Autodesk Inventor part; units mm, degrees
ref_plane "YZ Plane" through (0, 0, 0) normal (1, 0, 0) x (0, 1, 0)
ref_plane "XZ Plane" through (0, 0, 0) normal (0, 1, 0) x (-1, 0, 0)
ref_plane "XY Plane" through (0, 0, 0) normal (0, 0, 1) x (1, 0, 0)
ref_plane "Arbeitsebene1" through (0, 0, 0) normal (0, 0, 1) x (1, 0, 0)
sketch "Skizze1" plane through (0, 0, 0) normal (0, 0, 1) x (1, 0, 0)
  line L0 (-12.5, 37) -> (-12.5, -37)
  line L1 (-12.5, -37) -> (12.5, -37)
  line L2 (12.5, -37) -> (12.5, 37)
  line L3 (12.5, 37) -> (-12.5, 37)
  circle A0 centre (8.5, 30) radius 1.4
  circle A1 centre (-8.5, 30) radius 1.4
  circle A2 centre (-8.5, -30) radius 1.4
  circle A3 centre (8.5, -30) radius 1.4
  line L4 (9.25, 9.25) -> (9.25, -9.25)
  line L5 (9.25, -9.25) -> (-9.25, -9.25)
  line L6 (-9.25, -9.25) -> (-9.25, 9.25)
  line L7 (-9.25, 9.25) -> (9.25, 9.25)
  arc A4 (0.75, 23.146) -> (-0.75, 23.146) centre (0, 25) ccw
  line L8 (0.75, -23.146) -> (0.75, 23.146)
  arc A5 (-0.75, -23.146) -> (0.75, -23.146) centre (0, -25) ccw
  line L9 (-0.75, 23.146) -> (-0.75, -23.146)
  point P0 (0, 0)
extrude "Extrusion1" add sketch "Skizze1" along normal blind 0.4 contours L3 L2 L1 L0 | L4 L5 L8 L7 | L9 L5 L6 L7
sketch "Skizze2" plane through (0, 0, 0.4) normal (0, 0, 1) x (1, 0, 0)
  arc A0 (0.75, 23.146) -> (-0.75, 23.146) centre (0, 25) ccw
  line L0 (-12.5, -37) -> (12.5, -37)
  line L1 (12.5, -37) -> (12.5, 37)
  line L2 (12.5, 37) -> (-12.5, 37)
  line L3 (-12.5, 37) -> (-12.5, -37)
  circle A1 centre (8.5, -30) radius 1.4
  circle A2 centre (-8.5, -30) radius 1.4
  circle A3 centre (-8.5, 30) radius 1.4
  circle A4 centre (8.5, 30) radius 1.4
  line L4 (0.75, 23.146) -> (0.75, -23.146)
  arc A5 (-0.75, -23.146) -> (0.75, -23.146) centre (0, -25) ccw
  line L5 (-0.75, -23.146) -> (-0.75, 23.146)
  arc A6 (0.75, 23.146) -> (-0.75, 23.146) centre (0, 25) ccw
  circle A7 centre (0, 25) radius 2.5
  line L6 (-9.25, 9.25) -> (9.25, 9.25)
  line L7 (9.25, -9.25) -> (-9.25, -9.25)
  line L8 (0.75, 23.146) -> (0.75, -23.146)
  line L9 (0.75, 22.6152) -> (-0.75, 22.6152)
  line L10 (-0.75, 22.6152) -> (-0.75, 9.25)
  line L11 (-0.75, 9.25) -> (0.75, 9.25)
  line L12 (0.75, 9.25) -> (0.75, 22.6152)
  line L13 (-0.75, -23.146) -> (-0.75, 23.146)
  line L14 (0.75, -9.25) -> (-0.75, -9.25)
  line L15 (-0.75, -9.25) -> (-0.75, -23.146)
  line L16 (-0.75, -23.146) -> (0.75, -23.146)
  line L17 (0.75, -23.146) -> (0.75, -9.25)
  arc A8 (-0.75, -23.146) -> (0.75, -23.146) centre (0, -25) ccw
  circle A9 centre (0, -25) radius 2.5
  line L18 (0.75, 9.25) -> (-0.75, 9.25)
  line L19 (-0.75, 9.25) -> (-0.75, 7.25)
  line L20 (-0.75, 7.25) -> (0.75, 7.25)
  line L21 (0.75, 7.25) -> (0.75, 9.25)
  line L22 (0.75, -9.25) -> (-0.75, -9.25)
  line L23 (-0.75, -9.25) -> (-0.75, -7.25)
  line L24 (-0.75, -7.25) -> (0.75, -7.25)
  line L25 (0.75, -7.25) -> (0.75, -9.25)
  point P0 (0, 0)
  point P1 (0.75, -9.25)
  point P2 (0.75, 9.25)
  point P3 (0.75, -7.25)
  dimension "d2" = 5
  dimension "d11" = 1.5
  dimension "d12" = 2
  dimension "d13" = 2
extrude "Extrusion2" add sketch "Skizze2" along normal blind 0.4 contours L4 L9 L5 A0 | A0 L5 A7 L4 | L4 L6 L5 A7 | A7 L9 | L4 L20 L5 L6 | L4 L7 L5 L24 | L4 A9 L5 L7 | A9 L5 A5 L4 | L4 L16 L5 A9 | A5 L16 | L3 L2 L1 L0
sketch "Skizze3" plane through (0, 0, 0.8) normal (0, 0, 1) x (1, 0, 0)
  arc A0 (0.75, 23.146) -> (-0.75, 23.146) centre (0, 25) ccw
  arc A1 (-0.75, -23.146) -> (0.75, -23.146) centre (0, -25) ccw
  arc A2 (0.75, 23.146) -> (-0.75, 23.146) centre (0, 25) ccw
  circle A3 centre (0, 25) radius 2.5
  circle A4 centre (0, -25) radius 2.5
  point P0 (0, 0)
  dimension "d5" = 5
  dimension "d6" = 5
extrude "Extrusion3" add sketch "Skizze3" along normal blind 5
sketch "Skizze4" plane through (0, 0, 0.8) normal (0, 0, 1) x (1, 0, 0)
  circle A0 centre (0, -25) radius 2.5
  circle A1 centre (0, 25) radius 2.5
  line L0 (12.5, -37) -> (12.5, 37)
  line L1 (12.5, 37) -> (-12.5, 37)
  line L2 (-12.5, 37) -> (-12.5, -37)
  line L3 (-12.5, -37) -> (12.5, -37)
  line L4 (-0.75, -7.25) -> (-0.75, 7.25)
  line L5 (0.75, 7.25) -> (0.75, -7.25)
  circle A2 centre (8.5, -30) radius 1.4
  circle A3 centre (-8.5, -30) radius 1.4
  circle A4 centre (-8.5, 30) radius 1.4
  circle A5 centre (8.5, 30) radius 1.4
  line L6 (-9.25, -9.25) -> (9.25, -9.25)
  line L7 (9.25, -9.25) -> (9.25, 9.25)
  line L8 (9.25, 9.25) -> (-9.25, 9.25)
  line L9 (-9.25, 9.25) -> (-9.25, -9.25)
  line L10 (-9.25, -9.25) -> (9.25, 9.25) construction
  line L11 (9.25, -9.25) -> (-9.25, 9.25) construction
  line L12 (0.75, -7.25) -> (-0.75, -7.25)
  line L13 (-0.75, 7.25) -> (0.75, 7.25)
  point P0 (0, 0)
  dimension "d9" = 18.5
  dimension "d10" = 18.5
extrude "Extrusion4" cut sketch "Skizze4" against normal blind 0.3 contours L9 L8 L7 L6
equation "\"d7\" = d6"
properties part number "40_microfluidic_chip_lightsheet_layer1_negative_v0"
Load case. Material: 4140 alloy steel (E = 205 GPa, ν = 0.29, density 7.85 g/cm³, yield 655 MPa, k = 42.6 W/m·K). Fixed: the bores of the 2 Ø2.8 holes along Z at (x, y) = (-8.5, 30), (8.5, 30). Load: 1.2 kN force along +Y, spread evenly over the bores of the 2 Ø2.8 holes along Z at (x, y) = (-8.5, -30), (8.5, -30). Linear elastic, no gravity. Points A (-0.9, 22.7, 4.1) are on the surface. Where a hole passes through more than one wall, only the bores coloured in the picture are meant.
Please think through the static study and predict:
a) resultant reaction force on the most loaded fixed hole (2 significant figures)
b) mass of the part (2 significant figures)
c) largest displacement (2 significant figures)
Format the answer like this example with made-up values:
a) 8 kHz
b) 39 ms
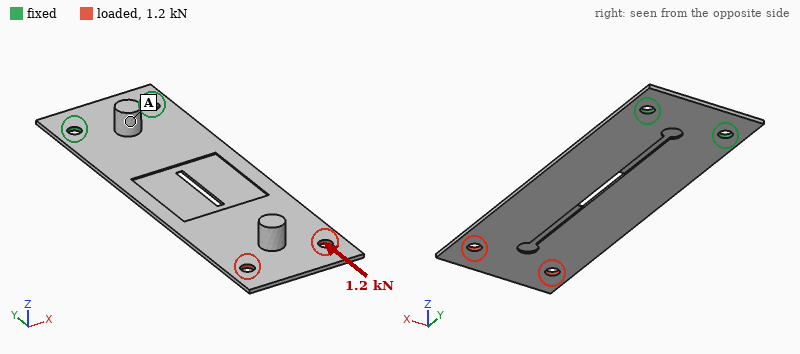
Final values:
a) 600 N
b) 12 g
c) 0.79 mm
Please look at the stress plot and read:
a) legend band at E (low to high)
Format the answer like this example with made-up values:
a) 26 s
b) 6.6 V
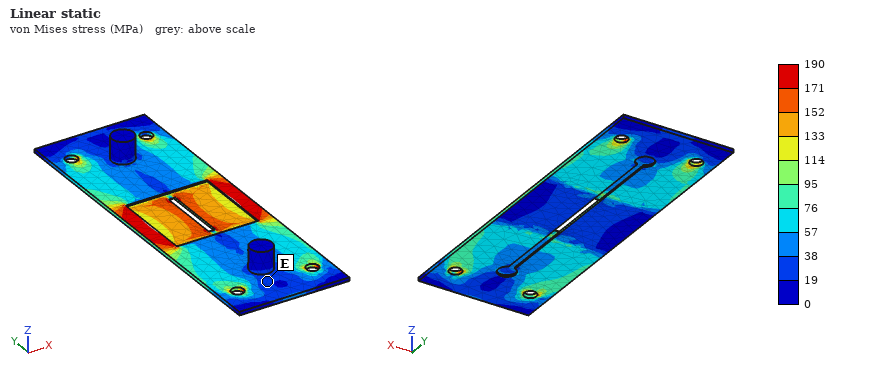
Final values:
a) 19 to 38 MPa
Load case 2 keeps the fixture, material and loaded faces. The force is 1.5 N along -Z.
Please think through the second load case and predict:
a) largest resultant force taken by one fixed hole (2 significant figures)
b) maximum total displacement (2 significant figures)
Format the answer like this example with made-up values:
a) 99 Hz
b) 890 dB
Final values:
a) 2.5 N
b) 0.72 mm
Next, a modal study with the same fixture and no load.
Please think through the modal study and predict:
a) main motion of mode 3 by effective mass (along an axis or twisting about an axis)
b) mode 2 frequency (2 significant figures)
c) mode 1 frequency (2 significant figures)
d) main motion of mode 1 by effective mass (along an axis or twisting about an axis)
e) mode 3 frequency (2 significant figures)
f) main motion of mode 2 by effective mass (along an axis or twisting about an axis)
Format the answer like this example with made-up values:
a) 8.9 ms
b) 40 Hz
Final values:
a) along Z
b) 710 Hz
c) 130 Hz
d) along Z
e) 880 Hz
f) twisting about Y
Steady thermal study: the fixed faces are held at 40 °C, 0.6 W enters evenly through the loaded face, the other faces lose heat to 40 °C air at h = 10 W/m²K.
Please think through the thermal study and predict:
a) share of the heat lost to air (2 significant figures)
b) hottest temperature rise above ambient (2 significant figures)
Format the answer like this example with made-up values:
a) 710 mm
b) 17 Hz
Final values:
a) 68 %
b) 25 K
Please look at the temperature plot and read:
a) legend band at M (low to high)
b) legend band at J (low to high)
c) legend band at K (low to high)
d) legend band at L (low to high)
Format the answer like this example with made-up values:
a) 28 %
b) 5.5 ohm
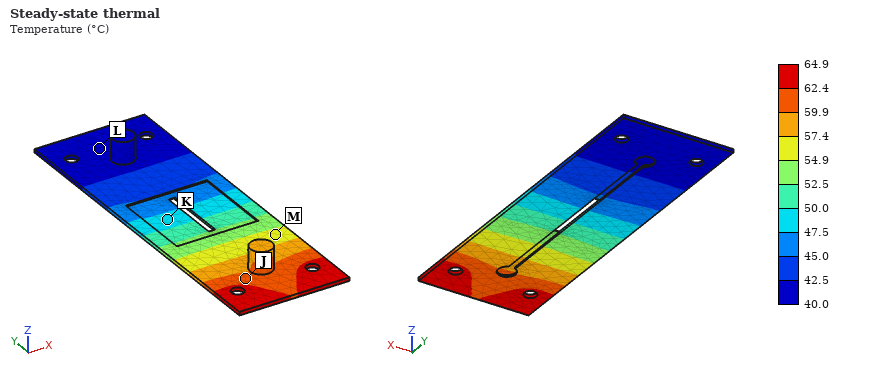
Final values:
a) 54.9 to 57.4 °C
b) 59.9 to 62.4 °C
c) 47.5 to 50.0 °C
d) 40.0 to 42.5 °C
